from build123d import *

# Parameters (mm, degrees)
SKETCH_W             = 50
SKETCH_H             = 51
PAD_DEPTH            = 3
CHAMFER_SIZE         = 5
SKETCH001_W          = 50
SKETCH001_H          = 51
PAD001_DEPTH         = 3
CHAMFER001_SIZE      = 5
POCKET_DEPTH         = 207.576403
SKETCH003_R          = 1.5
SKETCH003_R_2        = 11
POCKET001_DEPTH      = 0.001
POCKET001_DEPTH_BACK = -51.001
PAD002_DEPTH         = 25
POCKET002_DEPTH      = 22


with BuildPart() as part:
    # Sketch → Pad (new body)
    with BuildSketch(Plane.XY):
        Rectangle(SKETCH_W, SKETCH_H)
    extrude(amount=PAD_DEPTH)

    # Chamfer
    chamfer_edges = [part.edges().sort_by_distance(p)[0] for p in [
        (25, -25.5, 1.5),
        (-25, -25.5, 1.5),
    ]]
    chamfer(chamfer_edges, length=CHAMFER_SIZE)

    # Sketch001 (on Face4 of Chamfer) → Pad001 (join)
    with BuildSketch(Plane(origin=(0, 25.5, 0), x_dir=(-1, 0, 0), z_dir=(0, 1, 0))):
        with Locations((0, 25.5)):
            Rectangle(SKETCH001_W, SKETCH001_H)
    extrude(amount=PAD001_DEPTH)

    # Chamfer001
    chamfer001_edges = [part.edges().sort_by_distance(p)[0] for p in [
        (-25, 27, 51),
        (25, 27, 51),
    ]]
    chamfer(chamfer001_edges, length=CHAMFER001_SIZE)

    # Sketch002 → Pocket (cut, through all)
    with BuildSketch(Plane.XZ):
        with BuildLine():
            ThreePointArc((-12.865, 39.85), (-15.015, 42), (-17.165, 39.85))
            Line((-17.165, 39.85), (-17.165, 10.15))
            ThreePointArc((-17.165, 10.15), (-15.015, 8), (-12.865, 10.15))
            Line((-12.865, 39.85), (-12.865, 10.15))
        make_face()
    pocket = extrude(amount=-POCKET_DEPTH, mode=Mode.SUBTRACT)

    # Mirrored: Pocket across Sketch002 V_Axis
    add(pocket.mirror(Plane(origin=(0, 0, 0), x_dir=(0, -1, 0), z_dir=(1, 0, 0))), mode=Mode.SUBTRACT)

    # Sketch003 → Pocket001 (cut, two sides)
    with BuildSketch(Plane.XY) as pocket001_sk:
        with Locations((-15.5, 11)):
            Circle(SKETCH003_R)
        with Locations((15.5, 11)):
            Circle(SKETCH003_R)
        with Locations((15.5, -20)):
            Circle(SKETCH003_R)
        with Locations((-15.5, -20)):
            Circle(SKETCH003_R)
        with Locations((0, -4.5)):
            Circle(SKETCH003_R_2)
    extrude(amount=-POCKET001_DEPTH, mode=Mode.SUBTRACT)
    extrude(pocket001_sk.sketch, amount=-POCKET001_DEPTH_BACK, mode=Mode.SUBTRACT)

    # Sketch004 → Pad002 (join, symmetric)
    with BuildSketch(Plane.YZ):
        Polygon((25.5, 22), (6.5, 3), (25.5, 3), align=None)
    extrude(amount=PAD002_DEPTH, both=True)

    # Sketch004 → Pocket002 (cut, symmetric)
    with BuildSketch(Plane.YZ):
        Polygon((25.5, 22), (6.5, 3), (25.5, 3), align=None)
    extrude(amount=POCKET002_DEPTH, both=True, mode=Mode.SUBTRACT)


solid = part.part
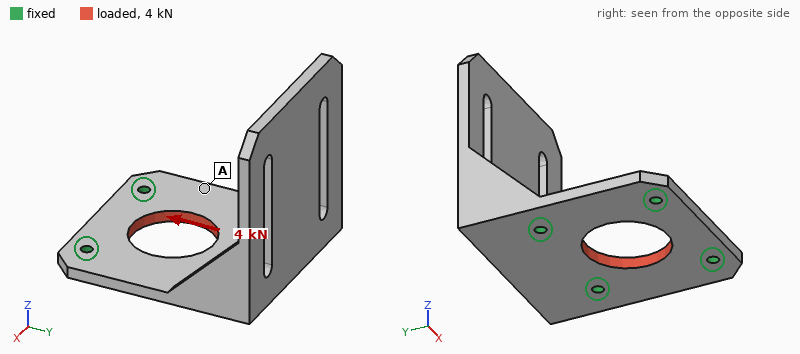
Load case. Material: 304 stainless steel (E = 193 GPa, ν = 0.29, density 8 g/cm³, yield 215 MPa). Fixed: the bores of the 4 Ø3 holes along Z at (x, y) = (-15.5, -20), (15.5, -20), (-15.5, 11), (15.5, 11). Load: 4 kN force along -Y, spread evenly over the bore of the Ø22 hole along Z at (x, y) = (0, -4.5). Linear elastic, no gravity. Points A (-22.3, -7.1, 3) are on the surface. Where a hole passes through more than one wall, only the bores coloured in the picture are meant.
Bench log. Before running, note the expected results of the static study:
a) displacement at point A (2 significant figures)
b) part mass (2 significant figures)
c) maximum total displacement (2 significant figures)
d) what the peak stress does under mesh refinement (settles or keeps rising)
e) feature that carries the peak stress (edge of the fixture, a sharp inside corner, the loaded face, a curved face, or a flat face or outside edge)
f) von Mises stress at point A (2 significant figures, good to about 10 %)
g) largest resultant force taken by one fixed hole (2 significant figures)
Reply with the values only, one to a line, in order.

0.73 µm
110 g
4.4 µm
keeps rising
edge of the fixture
6.2 MPa
1.0 kN
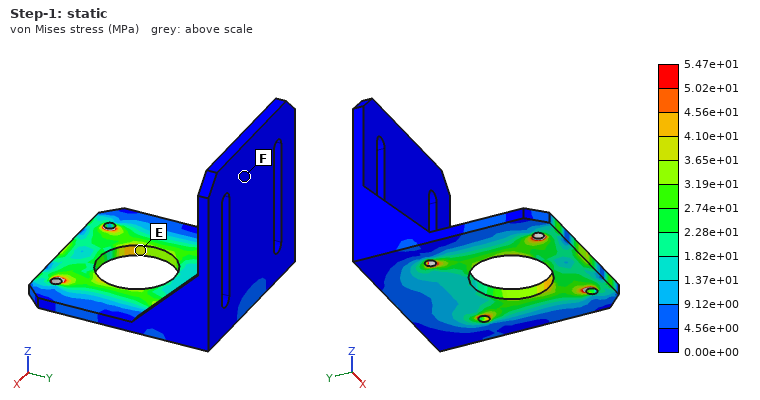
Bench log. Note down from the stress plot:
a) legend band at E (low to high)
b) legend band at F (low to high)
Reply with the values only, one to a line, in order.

3.65e+01 to 4.10e+01 MPa
0.00e+00 to 4.56e+00 MPa
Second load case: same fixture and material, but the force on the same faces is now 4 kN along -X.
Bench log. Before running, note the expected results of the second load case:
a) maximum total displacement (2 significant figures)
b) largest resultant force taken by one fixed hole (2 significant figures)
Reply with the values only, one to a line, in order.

3.4 µm
1.0 kN
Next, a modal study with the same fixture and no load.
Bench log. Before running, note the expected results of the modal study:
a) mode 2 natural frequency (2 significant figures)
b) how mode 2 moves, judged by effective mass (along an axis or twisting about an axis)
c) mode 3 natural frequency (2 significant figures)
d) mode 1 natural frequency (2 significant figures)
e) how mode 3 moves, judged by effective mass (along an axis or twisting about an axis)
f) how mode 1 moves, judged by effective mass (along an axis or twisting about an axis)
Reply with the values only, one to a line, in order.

1800 Hz
along X
3300 Hz
1000 Hz
along Z
along Y
